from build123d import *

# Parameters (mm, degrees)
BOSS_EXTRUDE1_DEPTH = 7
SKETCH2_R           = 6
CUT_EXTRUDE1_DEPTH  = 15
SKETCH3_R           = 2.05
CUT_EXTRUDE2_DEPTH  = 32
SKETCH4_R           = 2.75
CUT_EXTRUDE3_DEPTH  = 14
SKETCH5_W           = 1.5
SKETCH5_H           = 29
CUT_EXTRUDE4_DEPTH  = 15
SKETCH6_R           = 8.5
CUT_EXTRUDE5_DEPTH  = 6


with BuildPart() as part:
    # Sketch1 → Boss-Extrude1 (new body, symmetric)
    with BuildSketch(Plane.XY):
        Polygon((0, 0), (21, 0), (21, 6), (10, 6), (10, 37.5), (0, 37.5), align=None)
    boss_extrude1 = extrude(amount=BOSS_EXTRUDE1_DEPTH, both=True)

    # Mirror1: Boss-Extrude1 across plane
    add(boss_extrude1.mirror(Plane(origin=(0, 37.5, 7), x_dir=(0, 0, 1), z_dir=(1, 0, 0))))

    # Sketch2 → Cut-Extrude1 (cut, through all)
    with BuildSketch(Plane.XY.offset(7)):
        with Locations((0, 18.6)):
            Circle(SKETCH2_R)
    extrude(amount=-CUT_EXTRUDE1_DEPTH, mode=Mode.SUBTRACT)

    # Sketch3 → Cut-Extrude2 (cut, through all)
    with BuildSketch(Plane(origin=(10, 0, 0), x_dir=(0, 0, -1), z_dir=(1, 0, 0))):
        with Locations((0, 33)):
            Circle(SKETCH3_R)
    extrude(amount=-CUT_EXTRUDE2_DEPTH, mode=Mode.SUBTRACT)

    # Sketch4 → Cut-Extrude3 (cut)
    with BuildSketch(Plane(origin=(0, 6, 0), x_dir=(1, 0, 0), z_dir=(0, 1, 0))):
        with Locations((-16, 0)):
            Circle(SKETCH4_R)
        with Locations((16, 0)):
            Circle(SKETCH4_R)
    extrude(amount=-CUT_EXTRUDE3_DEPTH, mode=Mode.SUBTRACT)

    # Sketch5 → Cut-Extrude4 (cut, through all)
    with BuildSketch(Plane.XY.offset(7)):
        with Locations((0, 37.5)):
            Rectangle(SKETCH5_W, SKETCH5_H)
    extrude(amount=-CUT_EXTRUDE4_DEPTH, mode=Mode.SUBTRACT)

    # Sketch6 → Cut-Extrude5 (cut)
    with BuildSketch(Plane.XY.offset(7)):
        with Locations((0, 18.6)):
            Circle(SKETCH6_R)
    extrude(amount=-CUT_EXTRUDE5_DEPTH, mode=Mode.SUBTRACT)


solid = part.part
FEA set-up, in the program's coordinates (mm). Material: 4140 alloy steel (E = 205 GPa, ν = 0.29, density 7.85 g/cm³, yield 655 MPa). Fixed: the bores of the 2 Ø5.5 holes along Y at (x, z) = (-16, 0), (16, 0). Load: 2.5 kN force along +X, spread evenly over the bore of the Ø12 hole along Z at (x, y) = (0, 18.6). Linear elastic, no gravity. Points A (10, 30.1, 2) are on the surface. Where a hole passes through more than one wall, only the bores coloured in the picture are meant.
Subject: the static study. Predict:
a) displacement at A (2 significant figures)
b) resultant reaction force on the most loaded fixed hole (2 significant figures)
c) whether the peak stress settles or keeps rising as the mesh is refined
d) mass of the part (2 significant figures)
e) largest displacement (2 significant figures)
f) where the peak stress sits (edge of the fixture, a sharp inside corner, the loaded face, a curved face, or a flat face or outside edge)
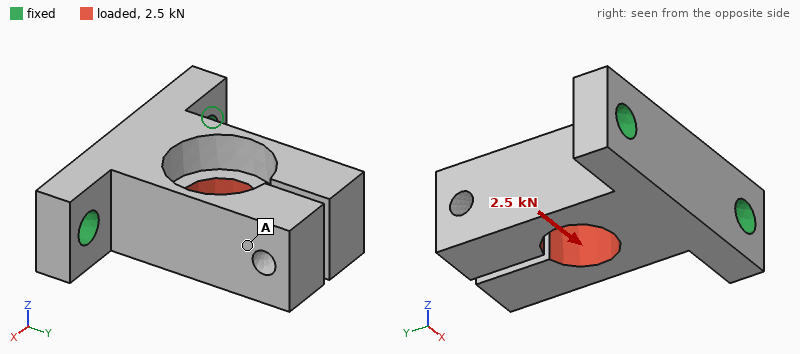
44 µm
2.0 kN
keeps rising
73 g
68 µm
a sharp inside corner
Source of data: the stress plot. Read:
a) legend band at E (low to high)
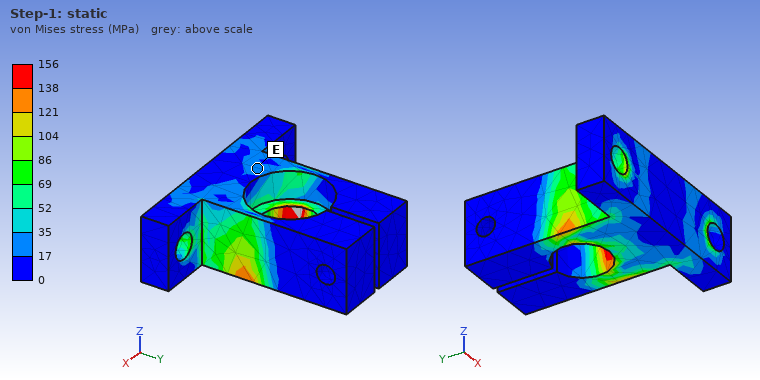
17 to 35 MPa
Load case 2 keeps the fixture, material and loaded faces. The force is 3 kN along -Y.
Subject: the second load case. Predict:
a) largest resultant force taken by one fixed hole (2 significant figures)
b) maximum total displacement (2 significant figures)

1.6 kN
54 µm
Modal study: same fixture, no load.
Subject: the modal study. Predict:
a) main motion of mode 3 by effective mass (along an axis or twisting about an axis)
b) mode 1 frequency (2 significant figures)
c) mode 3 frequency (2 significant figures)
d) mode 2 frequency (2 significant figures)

along Z
3300 Hz
4100 Hz
3300 Hz
